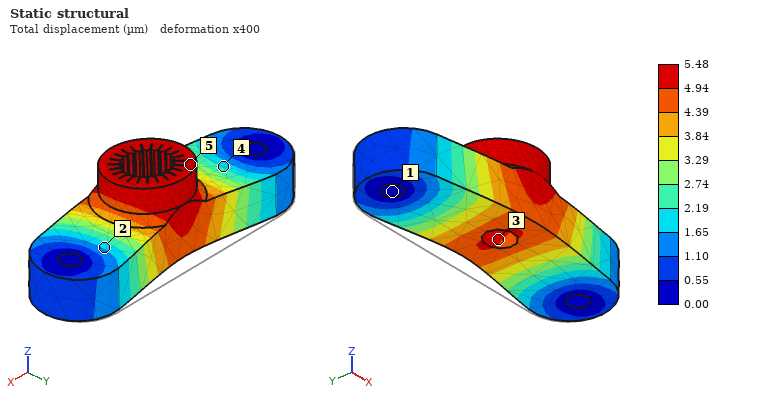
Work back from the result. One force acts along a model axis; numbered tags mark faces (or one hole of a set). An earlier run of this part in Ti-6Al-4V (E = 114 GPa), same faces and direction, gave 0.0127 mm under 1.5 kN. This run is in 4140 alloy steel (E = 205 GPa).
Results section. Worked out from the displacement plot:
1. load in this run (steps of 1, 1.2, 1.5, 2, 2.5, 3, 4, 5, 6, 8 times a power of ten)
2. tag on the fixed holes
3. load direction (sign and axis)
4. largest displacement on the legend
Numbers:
1.2 kN
1
-Y
5.48 µm
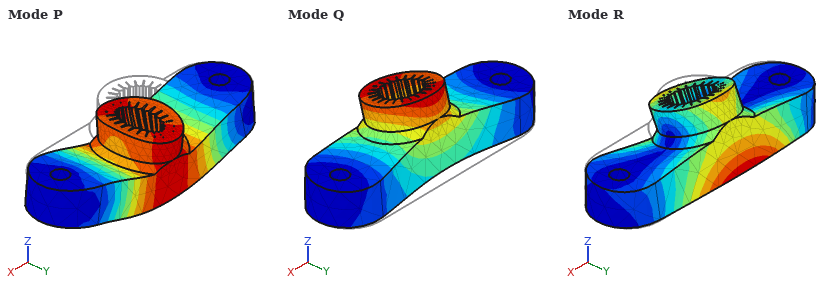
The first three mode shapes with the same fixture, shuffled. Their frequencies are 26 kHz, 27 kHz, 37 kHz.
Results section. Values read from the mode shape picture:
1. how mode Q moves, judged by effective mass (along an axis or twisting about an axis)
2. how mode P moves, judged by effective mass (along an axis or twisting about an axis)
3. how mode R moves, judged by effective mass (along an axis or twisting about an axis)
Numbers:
along Y
along Z
along Y
